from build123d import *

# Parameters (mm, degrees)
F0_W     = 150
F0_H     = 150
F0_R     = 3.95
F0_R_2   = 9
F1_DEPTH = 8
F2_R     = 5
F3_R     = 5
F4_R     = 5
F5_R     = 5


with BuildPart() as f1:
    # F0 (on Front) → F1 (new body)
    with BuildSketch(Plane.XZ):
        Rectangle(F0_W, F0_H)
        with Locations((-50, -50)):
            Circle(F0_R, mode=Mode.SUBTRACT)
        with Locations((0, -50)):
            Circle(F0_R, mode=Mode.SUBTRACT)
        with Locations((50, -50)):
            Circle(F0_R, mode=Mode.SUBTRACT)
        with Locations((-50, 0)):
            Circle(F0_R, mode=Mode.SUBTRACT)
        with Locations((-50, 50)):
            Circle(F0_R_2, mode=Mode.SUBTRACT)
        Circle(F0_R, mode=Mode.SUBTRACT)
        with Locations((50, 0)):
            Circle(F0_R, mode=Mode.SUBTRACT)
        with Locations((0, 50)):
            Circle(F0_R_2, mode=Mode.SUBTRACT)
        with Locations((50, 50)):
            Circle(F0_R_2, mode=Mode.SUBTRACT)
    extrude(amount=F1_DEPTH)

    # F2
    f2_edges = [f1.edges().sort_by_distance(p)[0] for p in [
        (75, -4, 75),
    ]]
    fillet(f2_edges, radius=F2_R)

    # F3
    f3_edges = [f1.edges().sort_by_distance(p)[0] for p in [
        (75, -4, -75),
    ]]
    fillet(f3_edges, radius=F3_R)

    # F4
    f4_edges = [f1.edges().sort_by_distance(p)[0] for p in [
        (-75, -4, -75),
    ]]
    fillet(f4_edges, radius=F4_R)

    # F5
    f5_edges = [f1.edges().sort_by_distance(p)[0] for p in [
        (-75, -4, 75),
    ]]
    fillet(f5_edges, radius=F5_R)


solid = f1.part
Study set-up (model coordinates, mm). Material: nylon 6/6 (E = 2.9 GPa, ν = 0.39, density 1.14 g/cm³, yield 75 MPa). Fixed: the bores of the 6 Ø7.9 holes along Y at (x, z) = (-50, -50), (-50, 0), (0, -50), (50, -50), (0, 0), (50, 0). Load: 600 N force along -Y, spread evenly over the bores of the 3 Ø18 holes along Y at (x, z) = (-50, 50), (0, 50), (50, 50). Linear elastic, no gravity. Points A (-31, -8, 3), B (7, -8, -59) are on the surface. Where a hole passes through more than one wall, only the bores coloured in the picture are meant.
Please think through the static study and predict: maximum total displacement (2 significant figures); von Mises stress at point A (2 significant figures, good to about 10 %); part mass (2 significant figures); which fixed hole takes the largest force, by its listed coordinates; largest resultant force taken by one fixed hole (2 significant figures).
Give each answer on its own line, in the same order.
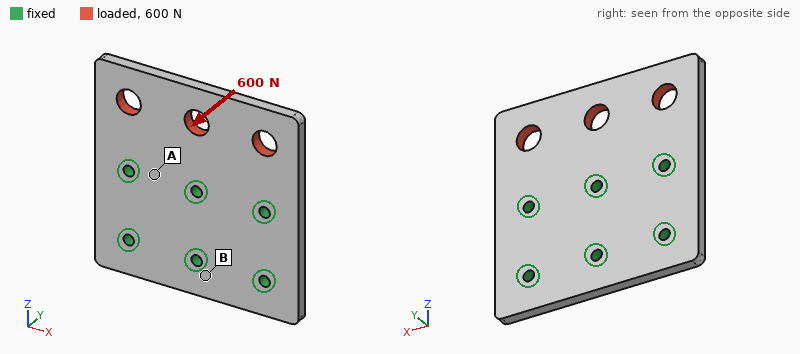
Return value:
2.4 mm
9.7 MPa
200 g
(0, 0)
300 N
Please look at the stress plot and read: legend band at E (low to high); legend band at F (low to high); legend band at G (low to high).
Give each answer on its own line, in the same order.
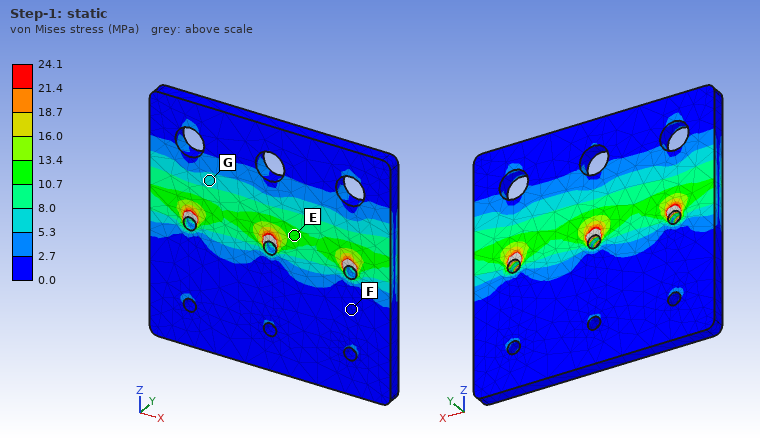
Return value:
10.7 to 13.4 MPa
0.0 to 2.7 MPa
5.3 to 8.0 MPa
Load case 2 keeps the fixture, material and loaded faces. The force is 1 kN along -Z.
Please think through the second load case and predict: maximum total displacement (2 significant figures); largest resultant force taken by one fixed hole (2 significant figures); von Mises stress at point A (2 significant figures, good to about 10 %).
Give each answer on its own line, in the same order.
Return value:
25 µm
280 N
0.47 MPa
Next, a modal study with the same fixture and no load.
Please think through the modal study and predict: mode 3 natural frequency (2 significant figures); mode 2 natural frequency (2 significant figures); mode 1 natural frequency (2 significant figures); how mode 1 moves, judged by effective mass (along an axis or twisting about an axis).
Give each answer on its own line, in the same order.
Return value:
970 Hz
550 Hz
380 Hz
along Y
